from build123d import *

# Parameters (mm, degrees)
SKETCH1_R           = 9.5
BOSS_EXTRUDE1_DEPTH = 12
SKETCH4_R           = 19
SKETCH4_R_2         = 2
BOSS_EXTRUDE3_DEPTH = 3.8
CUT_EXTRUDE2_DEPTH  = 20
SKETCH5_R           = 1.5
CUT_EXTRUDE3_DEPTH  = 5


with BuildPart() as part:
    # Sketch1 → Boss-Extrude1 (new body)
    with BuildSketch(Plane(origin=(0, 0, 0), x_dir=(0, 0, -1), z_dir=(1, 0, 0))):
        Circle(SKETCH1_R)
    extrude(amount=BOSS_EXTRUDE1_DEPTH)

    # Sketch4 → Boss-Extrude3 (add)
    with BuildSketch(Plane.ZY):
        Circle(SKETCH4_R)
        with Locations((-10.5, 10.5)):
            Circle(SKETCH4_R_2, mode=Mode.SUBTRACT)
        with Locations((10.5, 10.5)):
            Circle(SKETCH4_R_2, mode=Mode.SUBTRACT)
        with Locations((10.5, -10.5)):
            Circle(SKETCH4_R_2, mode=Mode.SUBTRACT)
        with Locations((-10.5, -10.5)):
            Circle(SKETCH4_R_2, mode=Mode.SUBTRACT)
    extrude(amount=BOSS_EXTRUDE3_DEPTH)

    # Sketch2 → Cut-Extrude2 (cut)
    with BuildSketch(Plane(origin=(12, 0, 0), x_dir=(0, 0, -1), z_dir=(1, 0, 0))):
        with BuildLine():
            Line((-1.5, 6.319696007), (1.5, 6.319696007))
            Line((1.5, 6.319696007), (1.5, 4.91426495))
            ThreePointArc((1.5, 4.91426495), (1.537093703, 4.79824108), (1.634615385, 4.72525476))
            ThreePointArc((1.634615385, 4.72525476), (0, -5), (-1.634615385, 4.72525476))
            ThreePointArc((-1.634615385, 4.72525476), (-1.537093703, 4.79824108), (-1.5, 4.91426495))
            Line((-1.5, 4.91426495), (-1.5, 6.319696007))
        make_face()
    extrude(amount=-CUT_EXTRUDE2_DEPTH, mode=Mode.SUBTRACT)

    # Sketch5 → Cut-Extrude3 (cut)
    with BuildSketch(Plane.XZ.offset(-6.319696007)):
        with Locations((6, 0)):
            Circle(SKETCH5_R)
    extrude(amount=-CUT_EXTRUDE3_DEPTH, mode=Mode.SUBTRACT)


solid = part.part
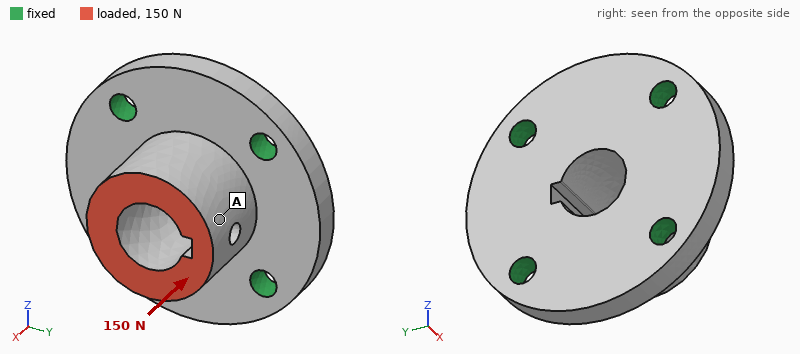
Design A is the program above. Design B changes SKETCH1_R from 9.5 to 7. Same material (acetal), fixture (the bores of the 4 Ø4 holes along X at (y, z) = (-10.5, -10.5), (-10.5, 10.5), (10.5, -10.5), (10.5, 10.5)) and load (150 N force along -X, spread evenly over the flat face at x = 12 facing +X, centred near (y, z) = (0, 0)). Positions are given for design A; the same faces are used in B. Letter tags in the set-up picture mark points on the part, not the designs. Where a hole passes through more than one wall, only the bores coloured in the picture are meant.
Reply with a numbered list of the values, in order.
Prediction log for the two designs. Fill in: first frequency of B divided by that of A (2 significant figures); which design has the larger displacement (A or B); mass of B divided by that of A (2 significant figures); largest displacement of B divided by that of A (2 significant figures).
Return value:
1. 0.96
2. B
3. 0.75
4. 2.4
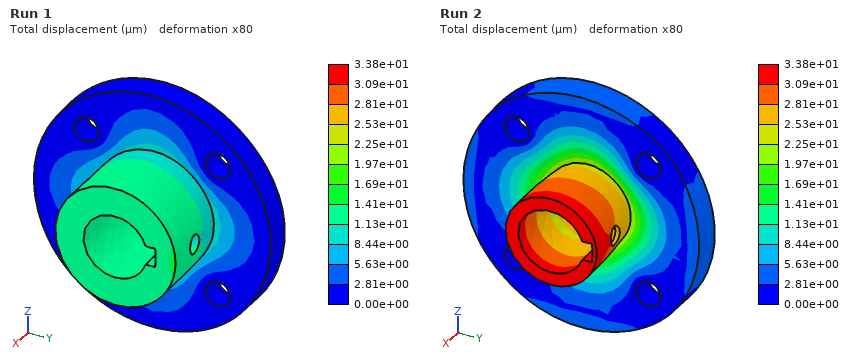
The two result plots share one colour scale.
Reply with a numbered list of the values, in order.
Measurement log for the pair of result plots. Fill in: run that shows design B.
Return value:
1. Run 2
